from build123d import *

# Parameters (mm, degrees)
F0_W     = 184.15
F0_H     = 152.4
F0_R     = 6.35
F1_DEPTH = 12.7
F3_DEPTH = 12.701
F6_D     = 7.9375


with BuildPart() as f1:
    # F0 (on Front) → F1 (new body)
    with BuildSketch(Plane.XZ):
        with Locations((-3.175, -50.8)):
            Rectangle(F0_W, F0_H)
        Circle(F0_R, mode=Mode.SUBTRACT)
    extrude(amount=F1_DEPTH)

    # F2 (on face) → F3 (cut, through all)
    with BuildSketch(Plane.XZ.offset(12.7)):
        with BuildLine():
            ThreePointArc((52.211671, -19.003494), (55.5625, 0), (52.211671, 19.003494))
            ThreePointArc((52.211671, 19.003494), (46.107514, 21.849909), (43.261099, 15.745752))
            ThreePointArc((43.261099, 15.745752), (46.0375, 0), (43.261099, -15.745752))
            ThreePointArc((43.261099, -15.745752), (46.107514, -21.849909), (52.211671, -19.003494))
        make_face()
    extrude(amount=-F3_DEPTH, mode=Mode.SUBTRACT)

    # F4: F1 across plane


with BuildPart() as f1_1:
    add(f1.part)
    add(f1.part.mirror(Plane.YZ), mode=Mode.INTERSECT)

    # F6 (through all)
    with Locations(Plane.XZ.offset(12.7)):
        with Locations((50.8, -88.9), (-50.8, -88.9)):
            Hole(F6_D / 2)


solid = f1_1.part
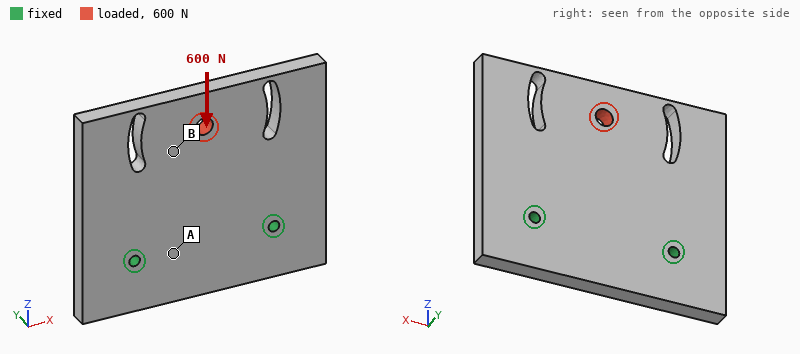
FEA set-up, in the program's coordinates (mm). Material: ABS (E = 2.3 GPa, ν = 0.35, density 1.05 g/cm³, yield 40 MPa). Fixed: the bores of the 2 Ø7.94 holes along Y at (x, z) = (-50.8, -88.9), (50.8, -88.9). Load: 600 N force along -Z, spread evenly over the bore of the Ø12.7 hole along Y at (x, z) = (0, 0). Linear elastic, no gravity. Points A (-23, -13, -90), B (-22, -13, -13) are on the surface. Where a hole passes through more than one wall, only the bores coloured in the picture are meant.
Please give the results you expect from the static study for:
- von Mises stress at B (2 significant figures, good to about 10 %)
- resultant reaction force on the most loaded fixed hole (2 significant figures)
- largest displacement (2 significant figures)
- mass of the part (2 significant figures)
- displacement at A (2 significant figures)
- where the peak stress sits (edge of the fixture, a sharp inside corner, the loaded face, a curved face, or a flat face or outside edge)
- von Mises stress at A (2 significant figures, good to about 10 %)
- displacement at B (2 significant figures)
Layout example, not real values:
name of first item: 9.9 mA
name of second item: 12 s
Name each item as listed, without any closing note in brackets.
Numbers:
von Mises stress at B: 0.59 MPa
resultant reaction force on the most loaded fixed hole: 310 N
largest displacement: 36 µm
mass of the part: 350 g
displacement at A: 8.7 µm
where the peak stress sits: the loaded face
von Mises stress at A: 0.24 MPa
displacement at B: 20 µm
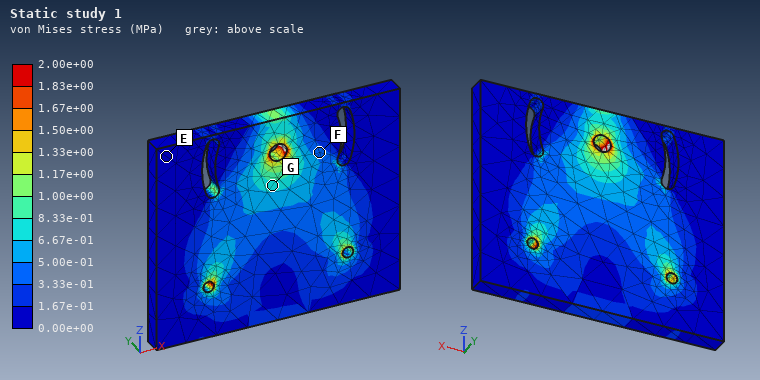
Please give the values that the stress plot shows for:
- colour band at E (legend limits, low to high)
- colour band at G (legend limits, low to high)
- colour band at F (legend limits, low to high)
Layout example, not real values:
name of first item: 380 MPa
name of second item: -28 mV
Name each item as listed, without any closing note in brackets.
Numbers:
colour band at E: 0.00e+00 to 1.67e-01 MPa
colour band at G: 6.67e-01 to 8.33e-01 MPa
colour band at F: 3.33e-01 to 5.00e-01 MPa
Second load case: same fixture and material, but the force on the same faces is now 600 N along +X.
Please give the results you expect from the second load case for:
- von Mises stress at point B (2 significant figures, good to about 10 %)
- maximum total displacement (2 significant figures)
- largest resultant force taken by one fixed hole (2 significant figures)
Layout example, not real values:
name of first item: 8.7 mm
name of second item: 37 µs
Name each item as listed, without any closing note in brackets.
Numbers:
von Mises stress at point B: 0.93 MPa
maximum total displacement: 86 µm
largest resultant force taken by one fixed hole: 590 N
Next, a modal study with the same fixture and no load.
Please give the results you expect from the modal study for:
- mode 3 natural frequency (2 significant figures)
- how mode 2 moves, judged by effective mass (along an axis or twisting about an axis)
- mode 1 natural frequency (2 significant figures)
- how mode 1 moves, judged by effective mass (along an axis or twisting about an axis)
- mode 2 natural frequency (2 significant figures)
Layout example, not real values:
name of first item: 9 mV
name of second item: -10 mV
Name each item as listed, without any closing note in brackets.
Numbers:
mode 3 natural frequency: 720 Hz
how mode 2 moves, judged by effective mass: twisting about Z
mode 1 natural frequency: 210 Hz
how mode 1 moves, judged by effective mass: along Y
mode 2 natural frequency: 370 Hz
